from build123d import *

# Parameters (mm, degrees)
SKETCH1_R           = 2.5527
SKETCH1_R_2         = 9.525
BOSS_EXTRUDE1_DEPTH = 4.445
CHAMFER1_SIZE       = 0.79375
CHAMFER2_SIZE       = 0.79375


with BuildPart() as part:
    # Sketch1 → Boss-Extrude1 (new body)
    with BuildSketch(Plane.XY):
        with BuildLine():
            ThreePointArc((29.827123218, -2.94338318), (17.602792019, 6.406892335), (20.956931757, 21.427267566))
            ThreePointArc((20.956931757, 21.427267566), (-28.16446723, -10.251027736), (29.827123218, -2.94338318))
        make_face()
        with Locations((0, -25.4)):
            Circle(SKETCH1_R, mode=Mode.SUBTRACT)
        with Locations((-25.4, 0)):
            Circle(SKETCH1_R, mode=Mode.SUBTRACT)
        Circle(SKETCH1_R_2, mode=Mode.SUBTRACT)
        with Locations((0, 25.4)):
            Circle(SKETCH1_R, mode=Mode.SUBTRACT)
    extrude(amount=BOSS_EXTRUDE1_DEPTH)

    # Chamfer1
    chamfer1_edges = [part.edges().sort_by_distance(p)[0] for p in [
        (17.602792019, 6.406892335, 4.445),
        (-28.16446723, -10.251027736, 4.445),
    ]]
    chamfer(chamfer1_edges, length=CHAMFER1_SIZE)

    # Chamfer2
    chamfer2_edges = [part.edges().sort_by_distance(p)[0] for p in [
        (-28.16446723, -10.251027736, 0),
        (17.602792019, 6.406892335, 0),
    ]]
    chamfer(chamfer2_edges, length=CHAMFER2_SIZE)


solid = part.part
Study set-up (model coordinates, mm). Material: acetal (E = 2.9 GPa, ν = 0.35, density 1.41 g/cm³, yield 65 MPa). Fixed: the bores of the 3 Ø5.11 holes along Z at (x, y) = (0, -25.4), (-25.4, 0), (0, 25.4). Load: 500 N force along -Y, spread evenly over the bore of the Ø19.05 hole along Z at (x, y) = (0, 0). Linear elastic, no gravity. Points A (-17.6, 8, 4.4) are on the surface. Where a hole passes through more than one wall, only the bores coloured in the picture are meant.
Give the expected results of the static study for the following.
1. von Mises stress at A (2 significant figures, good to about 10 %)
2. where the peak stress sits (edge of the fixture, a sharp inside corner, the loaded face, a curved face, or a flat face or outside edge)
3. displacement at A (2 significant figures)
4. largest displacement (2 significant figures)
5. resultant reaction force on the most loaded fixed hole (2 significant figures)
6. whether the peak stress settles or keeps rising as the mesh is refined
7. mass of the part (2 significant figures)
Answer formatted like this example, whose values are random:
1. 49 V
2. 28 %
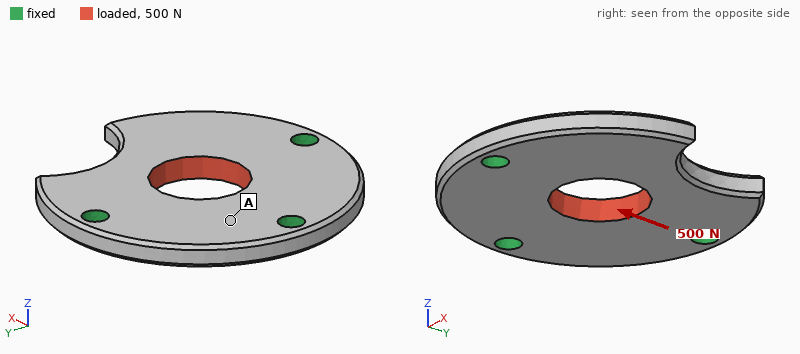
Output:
1. 0.89 MPa
2. edge of the fixture
3. 8.2 µm
4. 27 µm
5. 210 N
6. keeps rising
7. 14 g
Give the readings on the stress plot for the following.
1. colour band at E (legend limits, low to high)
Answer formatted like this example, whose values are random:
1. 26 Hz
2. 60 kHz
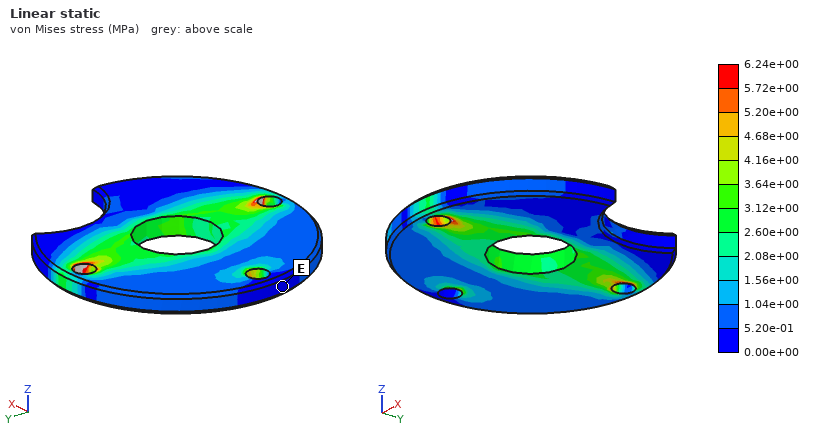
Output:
1. 0.00e+00 to 5.20e-01 MPa
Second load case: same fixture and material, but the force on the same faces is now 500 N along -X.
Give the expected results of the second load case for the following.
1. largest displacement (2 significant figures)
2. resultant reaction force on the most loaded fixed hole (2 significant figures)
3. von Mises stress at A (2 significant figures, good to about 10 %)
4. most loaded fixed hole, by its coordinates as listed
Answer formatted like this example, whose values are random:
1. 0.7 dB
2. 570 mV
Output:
1. 45 µm
2. 200 N
3. 2.1 MPa
4. (-25.4, 0)
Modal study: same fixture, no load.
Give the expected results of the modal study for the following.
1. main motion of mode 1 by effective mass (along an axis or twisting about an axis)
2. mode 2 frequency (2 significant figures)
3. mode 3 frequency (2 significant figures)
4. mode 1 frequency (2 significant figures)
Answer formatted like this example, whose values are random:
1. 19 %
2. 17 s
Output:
1. along Z
2. 3200 Hz
3. 4300 Hz
4. 1300 Hz
